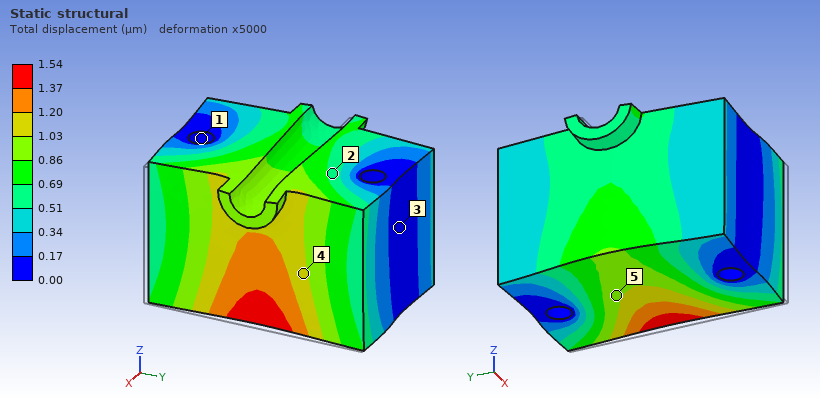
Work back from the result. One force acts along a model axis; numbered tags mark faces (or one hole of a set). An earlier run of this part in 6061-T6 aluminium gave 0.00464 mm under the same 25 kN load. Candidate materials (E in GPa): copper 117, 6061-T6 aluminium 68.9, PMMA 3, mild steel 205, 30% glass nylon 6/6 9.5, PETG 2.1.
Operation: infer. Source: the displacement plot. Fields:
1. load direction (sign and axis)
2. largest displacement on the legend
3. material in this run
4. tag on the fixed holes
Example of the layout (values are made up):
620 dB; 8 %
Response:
-X; 1.54 µm; mild steel; 1
